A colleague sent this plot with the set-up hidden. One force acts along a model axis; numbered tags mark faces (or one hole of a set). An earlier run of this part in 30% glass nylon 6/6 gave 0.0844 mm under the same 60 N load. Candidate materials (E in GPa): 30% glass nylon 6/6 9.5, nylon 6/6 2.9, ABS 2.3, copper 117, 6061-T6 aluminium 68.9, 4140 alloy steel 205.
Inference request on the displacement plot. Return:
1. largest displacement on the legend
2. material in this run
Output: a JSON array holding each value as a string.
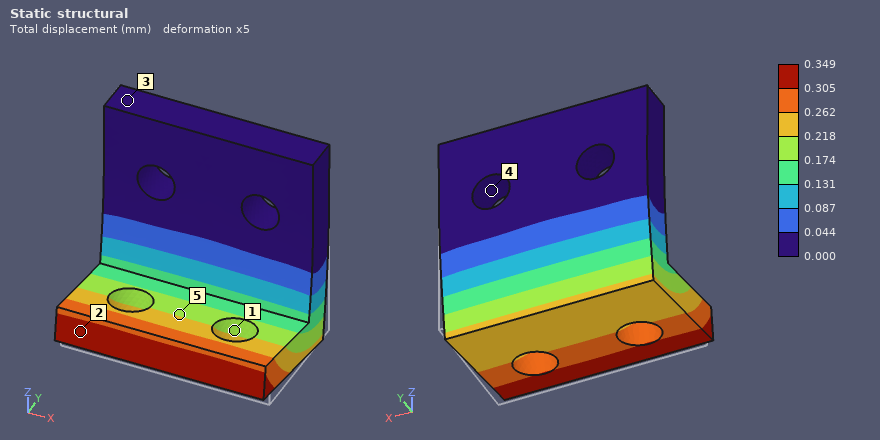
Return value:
["0.349 mm", "ABS"]
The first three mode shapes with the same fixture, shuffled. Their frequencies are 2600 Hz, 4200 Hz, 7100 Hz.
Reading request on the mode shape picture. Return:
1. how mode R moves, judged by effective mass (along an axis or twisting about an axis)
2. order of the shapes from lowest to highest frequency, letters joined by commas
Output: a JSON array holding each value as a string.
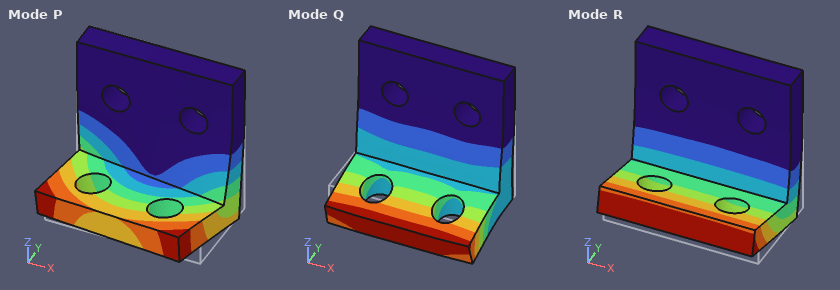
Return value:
["along Y", "R, P, Q"]
